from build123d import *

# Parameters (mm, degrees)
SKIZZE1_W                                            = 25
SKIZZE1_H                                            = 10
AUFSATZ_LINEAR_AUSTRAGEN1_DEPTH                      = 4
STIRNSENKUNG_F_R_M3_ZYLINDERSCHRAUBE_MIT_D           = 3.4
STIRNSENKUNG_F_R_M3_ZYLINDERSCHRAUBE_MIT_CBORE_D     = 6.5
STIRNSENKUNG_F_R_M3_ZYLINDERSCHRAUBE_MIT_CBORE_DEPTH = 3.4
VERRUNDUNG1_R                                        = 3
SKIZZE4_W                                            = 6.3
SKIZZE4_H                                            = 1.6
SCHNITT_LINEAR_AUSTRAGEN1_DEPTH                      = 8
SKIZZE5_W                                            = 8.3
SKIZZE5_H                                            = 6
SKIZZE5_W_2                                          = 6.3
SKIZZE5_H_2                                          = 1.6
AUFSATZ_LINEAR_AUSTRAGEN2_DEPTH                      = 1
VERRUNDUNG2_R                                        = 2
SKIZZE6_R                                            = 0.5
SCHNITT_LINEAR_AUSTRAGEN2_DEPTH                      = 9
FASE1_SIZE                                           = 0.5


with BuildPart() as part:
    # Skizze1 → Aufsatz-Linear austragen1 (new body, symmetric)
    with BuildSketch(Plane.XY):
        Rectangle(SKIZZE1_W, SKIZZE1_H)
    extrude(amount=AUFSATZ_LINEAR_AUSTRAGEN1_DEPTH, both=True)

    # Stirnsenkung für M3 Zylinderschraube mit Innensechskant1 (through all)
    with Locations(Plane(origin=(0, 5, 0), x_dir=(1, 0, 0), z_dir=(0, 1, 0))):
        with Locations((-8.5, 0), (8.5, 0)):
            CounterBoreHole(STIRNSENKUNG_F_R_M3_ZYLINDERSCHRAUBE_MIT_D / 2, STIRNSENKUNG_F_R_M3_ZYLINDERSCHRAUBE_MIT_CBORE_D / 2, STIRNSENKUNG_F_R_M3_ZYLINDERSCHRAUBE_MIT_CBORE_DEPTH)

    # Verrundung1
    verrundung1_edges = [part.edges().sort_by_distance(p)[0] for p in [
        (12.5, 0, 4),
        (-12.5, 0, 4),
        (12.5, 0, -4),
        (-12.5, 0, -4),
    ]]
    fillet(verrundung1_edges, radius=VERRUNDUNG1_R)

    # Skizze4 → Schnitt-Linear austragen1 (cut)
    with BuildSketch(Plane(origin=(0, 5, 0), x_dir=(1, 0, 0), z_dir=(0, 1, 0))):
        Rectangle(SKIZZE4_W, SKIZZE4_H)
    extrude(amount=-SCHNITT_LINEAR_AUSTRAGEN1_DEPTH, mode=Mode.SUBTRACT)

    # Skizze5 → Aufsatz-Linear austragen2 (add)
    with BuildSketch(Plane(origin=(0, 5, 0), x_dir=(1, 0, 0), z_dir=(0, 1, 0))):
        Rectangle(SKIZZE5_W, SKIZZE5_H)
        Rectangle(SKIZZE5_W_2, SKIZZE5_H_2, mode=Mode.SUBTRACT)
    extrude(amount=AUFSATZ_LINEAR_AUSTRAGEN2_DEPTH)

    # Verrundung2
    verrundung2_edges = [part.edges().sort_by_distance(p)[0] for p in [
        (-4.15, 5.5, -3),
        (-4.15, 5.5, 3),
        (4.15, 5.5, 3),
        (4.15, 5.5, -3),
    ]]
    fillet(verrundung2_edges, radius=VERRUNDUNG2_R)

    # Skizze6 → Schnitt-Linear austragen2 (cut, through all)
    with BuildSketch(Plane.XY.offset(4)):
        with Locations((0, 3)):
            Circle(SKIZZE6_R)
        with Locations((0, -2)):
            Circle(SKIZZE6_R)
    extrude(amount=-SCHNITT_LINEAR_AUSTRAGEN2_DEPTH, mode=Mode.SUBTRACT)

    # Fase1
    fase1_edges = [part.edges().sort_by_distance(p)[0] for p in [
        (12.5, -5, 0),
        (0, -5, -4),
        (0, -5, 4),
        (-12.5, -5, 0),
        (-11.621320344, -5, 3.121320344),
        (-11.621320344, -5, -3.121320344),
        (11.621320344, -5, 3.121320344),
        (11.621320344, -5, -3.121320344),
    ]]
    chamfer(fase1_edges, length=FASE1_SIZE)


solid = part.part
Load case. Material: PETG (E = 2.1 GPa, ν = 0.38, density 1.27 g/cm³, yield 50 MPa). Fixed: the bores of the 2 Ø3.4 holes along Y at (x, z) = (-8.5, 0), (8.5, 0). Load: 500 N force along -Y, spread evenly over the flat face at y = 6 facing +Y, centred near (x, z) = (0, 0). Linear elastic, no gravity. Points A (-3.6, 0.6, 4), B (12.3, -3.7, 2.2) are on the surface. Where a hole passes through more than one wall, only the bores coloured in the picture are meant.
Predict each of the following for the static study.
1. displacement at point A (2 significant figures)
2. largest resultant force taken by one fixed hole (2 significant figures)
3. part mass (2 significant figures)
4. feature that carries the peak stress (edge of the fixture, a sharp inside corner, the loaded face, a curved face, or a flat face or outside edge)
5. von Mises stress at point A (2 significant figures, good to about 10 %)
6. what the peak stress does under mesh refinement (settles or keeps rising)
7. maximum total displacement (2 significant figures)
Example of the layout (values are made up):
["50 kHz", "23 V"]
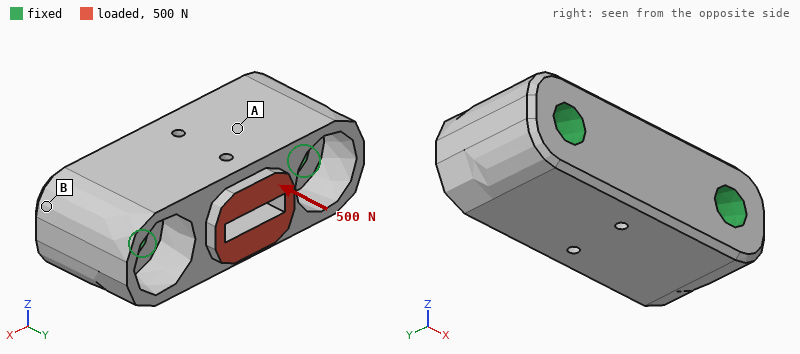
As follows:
["30 µm", "270 N", "1.9 g", "a sharp inside corner", "5.8 MPa", "keeps rising", "68 µm"]
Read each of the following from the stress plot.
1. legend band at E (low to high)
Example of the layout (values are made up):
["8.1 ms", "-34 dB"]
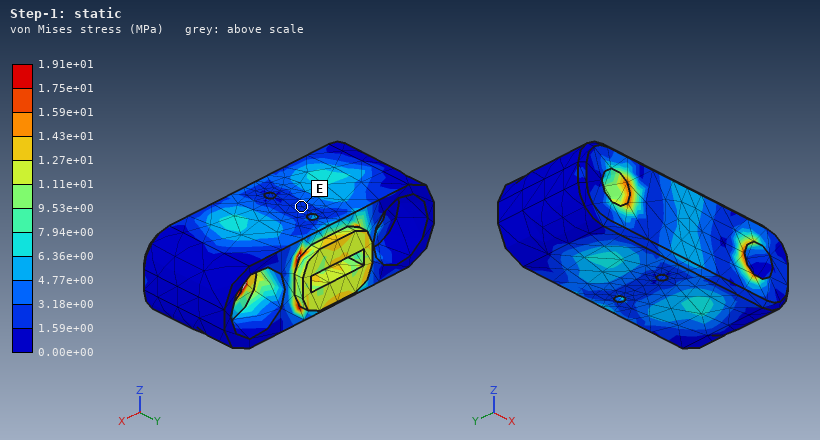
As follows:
["1.59e+00 to 3.18e+00 MPa"]
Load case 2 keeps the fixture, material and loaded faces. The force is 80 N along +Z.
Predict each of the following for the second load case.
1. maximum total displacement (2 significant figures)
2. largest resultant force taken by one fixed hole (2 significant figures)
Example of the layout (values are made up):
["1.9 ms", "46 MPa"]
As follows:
["64 µm", "40 N"]
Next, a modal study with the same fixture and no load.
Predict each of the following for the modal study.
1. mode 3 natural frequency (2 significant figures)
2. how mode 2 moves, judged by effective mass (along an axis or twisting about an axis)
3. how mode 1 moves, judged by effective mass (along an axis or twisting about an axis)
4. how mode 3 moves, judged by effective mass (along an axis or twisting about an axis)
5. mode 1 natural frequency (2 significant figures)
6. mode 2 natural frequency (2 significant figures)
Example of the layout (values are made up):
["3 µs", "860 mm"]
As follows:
["20 kHz", "along Y", "along Z", "along Z", "13 kHz", "19 kHz"]
